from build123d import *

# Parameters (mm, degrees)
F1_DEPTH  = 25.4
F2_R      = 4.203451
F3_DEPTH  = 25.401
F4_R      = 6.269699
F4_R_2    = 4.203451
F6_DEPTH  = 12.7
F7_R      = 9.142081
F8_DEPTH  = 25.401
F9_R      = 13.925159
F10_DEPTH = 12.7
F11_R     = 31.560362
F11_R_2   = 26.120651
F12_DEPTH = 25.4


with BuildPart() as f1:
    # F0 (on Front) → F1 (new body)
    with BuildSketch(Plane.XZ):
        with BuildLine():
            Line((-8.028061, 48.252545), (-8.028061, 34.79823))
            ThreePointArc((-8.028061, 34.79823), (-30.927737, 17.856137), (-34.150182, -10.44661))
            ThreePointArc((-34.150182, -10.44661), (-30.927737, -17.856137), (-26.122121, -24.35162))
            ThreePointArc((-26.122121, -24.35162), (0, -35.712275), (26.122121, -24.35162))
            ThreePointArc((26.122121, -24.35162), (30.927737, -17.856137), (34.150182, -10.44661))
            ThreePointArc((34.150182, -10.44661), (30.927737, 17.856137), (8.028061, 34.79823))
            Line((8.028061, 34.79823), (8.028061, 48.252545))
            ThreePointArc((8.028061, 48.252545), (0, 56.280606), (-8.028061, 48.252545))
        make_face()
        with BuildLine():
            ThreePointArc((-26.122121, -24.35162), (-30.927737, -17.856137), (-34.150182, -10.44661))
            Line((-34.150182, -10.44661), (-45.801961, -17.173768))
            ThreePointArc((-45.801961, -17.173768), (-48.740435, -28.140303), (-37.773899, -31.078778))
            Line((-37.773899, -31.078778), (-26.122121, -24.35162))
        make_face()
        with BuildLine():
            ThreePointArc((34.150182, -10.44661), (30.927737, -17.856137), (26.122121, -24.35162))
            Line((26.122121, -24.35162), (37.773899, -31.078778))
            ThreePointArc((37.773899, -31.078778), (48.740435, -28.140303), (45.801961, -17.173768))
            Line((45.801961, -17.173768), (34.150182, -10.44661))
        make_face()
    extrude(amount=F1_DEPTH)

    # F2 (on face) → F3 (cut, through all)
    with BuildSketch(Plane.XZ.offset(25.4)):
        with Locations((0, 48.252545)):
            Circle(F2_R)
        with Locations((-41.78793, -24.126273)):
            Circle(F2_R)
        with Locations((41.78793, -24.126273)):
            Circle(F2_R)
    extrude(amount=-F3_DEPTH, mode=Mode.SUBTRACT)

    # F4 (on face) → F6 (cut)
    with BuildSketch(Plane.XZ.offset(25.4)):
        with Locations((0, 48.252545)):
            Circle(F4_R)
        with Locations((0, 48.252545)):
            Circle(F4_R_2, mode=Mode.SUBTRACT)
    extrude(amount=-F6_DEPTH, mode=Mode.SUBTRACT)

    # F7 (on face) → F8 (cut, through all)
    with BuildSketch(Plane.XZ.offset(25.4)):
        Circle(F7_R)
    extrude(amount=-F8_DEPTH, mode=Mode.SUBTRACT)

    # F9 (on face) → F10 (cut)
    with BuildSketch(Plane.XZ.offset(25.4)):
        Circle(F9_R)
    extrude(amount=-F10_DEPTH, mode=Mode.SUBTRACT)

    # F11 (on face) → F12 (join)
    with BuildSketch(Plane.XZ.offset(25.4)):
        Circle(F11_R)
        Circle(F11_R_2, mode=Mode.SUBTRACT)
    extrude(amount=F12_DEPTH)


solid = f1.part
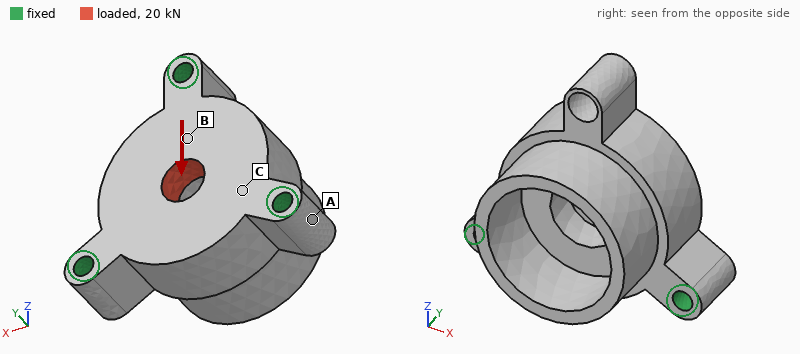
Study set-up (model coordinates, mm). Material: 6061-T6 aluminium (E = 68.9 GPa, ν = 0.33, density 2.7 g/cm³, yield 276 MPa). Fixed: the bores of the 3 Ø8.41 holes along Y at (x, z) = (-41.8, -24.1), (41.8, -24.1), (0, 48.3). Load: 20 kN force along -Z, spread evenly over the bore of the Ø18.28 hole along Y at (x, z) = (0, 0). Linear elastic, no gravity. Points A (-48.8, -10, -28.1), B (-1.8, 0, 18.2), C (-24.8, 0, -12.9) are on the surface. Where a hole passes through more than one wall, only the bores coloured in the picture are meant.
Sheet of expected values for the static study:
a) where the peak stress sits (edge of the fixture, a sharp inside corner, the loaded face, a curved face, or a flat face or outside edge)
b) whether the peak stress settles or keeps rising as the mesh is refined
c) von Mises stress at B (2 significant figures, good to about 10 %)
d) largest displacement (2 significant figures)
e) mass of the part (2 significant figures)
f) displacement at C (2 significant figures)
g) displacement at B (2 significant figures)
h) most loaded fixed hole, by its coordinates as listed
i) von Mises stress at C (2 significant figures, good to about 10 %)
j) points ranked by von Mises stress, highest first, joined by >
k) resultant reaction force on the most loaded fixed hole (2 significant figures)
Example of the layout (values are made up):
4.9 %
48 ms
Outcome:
edge of the fixture
keeps rising
37 MPa
28 µm
360 g
14 µm
13 µm
(0, 48.3)
17 MPa
B > C > A
7.9 kN
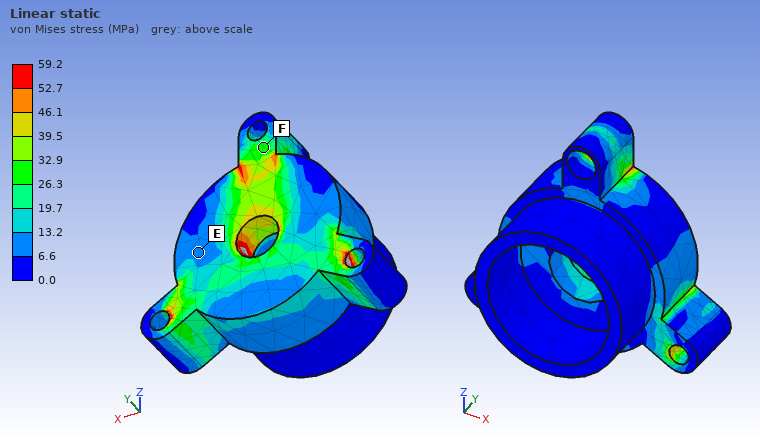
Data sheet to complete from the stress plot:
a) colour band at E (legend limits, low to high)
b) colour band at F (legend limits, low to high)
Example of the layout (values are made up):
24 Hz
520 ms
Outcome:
6.6 to 13.2 MPa
26.3 to 32.9 MPa
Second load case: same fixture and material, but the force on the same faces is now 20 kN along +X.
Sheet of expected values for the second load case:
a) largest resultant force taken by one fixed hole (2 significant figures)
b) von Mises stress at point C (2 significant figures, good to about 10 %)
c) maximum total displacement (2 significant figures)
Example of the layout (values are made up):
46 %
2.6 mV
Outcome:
9.1 kN
30 MPa
24 µm
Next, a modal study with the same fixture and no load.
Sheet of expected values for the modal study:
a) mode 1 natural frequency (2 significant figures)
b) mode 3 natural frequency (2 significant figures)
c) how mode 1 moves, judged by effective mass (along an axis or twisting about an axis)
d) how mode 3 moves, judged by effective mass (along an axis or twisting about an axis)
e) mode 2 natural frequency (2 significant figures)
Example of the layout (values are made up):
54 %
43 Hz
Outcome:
7300 Hz
8700 Hz
along X
along Y
7700 Hz
